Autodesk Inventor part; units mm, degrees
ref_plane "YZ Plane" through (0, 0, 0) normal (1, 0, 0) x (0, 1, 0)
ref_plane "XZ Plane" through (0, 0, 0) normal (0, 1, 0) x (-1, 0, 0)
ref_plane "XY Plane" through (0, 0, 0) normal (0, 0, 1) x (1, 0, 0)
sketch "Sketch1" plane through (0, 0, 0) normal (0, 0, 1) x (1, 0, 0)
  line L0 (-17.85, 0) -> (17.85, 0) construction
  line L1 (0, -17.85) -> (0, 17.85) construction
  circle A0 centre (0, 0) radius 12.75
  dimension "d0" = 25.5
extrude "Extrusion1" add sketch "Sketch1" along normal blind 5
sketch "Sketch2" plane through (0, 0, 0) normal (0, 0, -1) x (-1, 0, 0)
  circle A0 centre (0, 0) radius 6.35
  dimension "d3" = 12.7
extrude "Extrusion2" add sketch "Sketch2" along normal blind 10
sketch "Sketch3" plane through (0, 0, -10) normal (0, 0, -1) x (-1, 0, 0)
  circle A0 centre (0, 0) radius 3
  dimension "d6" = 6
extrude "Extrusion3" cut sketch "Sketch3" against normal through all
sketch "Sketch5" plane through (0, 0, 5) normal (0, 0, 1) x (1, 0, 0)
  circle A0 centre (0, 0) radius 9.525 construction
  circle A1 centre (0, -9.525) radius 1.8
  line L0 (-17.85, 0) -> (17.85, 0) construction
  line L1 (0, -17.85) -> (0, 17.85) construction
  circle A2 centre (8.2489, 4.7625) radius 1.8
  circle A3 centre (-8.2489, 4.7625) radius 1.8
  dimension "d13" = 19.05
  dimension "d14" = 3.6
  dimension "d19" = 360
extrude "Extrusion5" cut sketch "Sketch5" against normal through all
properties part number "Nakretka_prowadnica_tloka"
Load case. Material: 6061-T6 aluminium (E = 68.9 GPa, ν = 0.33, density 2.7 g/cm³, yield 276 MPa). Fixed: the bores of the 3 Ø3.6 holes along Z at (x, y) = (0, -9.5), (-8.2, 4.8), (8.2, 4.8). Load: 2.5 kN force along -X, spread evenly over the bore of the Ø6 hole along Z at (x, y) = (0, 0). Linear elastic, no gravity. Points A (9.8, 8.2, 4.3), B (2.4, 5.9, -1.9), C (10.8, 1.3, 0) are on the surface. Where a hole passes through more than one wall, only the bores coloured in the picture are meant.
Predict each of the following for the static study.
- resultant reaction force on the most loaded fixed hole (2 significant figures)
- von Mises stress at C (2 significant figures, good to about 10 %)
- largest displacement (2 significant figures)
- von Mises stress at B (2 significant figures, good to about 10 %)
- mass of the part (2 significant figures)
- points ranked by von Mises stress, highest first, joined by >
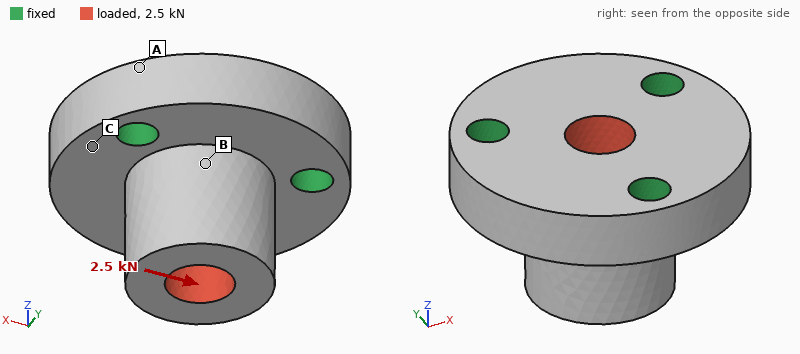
1.1 kN
16 MPa
17 µm
33 MPa
8.8 g
B > C > A
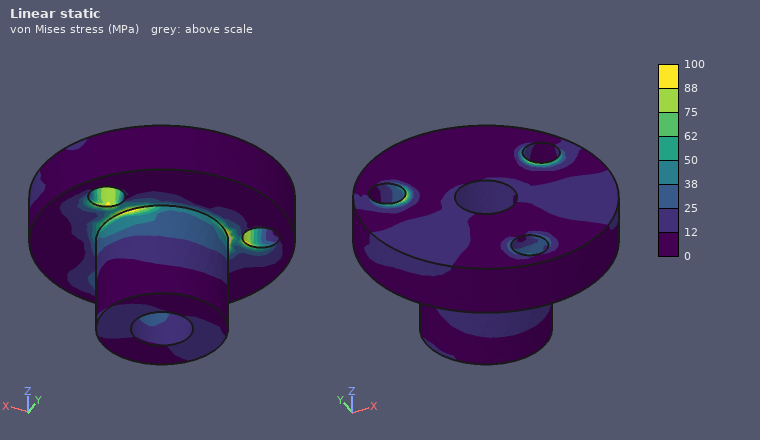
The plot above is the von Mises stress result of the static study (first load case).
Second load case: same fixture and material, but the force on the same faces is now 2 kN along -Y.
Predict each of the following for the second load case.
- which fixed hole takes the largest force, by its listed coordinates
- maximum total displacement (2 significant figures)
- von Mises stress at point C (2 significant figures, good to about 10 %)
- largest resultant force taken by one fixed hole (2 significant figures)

(0, -9.5)
13 µm
8.2 MPa
1000 N
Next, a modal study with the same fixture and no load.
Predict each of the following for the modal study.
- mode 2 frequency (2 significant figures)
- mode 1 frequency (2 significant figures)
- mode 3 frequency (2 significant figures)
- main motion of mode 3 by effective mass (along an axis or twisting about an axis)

35 kHz
35 kHz
51 kHz
along Z
